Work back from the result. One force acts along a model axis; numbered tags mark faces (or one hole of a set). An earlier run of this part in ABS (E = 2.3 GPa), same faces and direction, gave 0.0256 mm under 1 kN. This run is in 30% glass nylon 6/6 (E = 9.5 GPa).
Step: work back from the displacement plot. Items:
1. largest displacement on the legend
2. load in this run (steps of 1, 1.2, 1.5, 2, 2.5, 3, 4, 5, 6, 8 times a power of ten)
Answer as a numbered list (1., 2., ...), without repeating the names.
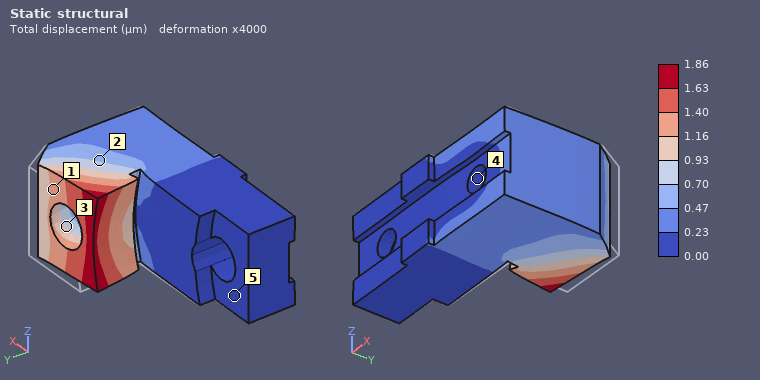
1. 1.86 µm
2. 300 N
